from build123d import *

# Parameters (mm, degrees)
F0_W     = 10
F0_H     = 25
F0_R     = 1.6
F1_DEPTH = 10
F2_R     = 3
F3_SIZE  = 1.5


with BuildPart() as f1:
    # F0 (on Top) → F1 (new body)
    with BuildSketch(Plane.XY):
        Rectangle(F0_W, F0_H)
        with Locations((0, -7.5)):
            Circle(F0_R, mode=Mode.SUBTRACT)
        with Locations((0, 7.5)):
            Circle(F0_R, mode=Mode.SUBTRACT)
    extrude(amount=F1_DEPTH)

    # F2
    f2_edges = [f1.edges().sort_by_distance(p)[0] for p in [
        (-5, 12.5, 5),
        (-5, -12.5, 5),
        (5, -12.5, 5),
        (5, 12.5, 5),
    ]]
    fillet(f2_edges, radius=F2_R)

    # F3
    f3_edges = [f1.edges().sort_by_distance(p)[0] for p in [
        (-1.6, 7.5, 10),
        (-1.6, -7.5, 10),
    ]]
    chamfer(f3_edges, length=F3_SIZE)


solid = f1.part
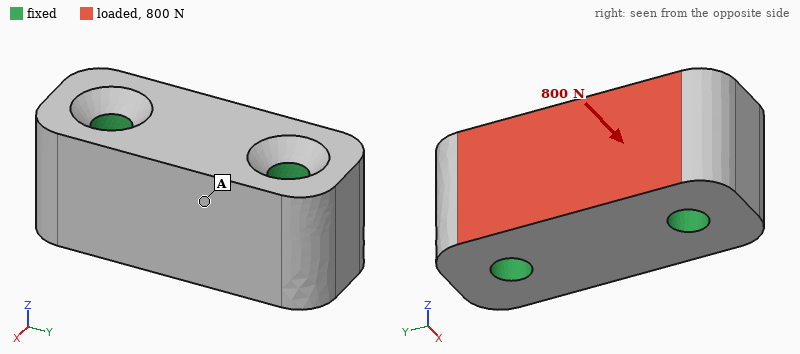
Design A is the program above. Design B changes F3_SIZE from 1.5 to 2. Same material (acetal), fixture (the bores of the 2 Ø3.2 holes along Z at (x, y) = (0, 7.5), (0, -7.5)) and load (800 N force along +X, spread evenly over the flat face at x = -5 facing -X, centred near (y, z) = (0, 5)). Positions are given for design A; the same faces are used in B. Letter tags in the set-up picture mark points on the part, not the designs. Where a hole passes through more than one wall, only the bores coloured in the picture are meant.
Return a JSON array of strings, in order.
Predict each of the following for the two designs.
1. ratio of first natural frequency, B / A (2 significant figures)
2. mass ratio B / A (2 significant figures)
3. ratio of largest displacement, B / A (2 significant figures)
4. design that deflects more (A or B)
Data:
["0.94", "0.99", "1.1", "B"]
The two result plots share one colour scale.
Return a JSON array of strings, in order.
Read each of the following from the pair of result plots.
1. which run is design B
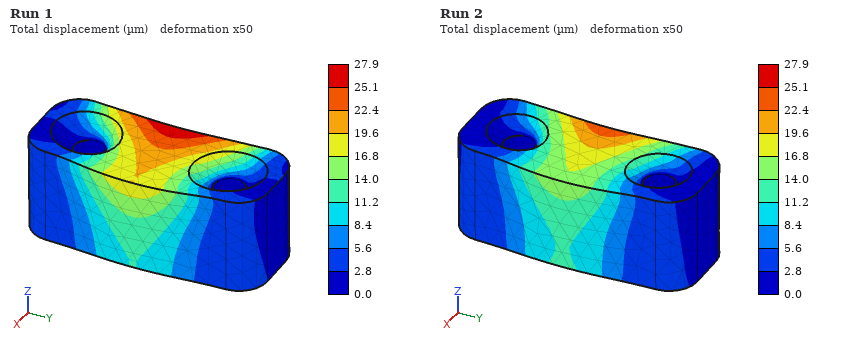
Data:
["Run 1"]
